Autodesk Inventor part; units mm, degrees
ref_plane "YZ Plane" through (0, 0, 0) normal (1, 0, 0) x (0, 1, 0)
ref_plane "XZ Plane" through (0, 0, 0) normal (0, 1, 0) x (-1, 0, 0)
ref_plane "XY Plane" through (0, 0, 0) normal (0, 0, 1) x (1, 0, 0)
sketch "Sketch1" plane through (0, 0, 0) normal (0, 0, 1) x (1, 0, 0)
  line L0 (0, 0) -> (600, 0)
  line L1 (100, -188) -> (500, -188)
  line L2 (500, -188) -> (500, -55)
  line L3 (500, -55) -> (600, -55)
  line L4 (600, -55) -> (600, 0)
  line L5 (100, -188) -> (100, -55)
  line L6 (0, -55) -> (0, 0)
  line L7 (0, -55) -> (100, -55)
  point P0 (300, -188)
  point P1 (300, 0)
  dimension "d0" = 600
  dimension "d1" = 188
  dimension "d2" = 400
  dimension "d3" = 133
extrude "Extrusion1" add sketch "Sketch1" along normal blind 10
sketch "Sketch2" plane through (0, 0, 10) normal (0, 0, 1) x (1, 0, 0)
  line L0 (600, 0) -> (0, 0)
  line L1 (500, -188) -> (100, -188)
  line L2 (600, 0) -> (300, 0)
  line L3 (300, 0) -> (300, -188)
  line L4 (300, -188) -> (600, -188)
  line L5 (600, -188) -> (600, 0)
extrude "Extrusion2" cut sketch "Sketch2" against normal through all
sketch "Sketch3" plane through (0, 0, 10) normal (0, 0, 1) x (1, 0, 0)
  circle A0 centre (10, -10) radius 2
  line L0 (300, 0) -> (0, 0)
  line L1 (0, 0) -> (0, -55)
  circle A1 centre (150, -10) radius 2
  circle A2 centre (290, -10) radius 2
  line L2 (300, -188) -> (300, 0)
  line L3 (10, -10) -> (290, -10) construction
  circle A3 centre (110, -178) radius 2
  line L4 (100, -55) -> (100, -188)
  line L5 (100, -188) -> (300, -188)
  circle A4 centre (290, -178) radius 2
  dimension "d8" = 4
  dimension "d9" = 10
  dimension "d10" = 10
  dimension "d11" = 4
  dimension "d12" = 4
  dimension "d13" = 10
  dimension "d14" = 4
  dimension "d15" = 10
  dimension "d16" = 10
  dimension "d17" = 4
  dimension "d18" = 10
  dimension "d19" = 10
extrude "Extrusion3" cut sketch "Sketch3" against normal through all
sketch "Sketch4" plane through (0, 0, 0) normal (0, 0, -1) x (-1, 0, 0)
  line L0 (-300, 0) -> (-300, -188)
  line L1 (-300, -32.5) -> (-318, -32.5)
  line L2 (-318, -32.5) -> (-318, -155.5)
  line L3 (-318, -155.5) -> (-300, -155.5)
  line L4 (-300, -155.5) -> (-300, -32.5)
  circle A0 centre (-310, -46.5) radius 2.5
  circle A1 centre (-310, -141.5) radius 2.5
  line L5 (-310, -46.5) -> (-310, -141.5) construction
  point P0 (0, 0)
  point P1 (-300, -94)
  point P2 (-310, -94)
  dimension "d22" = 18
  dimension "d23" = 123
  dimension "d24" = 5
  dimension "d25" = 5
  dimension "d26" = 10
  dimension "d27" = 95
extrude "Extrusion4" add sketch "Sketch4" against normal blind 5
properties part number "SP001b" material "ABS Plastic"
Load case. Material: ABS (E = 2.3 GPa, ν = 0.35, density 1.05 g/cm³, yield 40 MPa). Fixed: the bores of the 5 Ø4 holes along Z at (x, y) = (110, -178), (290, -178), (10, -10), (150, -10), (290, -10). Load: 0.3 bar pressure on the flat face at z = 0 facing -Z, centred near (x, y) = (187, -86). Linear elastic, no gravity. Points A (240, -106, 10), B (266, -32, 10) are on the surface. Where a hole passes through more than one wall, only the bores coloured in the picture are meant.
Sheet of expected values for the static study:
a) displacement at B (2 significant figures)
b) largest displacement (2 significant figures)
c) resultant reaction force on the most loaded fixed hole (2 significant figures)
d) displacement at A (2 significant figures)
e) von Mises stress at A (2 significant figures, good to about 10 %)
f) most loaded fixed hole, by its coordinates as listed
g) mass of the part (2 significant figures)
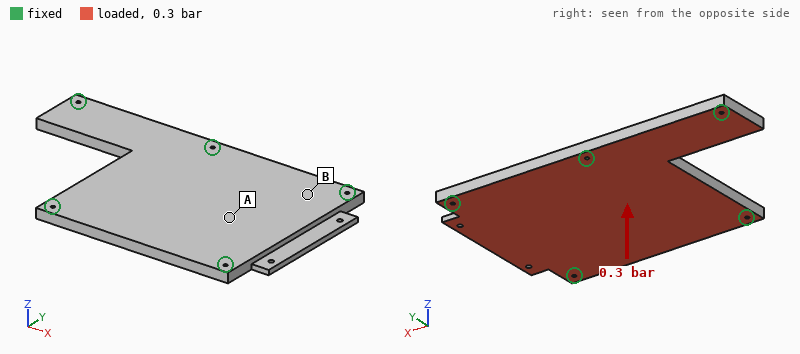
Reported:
0.38 mm
1.1 mm
400 N
1.0 mm
3.2 MPa
(150, -10)
460 g
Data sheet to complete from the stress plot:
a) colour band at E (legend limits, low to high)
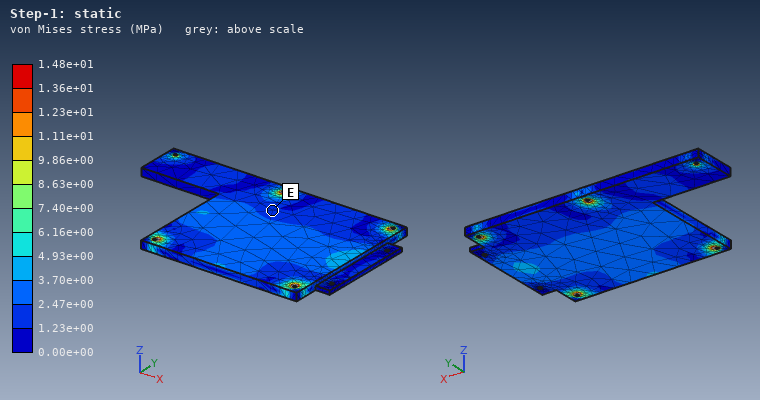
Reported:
1.23e+00 to 2.47e+00 MPa
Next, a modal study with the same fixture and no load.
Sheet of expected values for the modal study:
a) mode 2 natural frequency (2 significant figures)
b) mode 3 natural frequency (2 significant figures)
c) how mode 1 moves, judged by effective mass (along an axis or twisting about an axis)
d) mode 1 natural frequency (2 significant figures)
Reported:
450 Hz
480 Hz
along Z
310 Hz
